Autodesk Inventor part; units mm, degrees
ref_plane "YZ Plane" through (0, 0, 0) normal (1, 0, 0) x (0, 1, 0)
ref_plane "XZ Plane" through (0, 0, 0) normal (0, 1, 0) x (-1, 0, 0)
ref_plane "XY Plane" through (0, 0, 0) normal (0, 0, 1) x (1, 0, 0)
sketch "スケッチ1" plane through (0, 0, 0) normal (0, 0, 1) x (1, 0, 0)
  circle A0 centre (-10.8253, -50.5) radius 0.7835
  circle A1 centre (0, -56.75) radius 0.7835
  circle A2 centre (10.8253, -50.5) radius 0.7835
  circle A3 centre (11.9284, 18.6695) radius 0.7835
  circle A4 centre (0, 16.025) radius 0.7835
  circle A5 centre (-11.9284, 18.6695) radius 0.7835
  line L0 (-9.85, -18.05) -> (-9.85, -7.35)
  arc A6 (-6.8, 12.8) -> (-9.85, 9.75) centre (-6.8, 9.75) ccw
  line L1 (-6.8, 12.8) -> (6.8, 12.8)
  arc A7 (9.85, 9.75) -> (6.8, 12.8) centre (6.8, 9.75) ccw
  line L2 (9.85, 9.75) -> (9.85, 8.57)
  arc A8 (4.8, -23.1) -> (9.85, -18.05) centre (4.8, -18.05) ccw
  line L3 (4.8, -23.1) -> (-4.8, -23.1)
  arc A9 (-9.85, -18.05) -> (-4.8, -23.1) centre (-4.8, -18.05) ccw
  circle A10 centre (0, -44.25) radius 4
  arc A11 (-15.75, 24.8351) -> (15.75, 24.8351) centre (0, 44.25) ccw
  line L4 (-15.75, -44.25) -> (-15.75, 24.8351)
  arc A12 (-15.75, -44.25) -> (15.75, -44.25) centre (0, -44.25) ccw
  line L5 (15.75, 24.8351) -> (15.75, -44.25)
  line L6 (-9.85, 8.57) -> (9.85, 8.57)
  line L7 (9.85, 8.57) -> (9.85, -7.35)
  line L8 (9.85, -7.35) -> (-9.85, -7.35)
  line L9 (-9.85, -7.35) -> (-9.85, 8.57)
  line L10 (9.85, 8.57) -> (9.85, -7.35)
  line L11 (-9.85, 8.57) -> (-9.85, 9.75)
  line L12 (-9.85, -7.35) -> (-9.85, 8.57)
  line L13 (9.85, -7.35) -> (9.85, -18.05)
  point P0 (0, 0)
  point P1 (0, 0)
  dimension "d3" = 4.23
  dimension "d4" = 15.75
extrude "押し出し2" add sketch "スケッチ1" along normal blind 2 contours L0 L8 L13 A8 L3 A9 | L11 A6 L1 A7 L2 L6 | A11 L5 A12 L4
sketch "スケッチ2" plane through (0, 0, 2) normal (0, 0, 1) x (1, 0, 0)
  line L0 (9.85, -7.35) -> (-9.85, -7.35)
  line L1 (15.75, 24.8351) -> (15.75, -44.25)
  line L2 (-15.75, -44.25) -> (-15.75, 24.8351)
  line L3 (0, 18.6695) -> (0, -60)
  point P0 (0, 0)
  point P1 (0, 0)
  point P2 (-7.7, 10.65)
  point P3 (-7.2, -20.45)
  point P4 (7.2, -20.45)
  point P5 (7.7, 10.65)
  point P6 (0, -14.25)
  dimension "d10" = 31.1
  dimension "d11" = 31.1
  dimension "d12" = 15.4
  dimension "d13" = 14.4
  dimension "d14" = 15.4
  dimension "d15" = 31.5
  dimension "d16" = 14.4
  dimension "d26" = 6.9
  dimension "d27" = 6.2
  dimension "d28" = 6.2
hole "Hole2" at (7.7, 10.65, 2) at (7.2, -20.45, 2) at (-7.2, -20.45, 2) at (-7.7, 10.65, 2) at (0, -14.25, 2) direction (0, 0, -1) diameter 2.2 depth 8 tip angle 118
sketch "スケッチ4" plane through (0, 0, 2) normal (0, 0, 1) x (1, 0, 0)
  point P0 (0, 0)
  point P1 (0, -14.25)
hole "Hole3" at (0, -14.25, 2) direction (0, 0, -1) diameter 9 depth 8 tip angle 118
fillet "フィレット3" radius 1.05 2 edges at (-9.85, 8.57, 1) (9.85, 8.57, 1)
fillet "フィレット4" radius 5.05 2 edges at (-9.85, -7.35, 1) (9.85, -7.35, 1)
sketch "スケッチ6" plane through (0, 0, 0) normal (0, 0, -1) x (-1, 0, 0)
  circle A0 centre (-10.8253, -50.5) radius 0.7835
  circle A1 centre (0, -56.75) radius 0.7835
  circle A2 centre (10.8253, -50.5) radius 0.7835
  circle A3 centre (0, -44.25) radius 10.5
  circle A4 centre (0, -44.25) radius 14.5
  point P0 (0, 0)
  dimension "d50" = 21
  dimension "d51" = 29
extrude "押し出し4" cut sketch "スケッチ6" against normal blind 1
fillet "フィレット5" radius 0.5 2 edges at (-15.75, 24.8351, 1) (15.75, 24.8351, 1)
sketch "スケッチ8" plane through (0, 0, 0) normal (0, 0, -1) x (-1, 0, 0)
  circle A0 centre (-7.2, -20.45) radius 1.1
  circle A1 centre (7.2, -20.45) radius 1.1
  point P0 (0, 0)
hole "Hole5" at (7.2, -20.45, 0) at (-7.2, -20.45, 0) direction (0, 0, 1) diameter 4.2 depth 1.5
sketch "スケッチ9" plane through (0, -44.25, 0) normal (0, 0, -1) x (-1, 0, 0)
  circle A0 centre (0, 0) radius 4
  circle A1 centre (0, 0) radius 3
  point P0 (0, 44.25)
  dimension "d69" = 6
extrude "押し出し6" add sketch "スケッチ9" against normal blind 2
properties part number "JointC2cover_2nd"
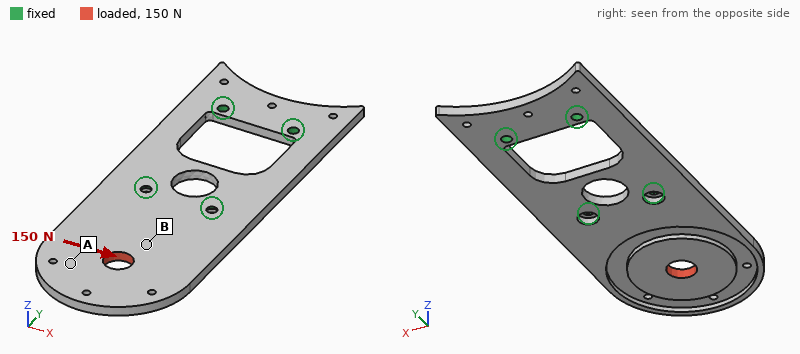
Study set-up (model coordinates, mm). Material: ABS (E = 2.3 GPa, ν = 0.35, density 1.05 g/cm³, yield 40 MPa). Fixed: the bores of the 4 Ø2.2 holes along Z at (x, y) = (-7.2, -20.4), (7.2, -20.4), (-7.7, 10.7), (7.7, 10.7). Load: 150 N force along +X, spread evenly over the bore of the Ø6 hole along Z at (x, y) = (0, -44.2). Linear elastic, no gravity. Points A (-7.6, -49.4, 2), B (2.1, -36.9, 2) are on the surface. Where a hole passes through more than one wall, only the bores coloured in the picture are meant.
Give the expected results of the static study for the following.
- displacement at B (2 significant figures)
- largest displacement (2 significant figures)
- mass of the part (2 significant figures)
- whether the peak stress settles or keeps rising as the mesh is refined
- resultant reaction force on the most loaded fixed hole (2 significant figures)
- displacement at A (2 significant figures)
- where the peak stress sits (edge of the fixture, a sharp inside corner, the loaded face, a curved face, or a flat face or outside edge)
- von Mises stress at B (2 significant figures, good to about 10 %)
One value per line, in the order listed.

0.21 mm
0.49 mm
3.9 g
keeps rising
160 N
0.38 mm
edge of the fixture
7.7 MPa
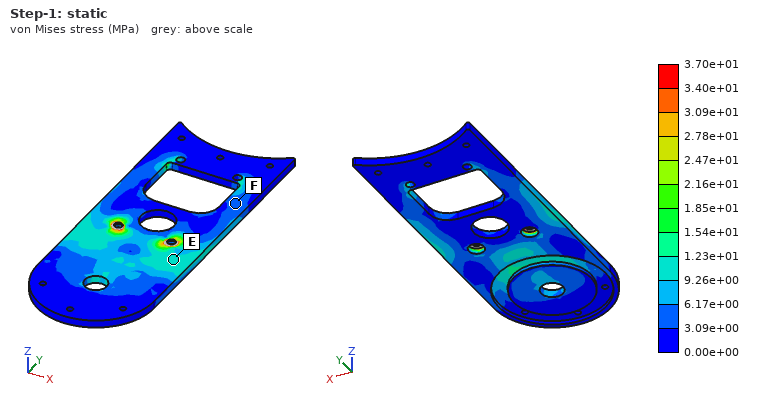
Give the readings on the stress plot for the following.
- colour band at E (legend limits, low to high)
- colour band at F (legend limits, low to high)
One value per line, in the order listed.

9.26e+00 to 1.23e+01 MPa
3.09e+00 to 6.17e+00 MPa
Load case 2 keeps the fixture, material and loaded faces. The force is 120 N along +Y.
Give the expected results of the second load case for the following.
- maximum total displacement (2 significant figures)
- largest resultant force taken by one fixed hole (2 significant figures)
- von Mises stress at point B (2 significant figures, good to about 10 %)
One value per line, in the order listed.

1.1 mm
47 N
2.8 MPa
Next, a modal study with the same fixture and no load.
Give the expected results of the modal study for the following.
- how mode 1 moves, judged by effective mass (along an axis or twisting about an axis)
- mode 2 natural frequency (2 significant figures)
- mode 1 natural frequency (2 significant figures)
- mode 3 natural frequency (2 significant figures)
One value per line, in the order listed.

along Z
910 Hz
290 Hz
1500 Hz
